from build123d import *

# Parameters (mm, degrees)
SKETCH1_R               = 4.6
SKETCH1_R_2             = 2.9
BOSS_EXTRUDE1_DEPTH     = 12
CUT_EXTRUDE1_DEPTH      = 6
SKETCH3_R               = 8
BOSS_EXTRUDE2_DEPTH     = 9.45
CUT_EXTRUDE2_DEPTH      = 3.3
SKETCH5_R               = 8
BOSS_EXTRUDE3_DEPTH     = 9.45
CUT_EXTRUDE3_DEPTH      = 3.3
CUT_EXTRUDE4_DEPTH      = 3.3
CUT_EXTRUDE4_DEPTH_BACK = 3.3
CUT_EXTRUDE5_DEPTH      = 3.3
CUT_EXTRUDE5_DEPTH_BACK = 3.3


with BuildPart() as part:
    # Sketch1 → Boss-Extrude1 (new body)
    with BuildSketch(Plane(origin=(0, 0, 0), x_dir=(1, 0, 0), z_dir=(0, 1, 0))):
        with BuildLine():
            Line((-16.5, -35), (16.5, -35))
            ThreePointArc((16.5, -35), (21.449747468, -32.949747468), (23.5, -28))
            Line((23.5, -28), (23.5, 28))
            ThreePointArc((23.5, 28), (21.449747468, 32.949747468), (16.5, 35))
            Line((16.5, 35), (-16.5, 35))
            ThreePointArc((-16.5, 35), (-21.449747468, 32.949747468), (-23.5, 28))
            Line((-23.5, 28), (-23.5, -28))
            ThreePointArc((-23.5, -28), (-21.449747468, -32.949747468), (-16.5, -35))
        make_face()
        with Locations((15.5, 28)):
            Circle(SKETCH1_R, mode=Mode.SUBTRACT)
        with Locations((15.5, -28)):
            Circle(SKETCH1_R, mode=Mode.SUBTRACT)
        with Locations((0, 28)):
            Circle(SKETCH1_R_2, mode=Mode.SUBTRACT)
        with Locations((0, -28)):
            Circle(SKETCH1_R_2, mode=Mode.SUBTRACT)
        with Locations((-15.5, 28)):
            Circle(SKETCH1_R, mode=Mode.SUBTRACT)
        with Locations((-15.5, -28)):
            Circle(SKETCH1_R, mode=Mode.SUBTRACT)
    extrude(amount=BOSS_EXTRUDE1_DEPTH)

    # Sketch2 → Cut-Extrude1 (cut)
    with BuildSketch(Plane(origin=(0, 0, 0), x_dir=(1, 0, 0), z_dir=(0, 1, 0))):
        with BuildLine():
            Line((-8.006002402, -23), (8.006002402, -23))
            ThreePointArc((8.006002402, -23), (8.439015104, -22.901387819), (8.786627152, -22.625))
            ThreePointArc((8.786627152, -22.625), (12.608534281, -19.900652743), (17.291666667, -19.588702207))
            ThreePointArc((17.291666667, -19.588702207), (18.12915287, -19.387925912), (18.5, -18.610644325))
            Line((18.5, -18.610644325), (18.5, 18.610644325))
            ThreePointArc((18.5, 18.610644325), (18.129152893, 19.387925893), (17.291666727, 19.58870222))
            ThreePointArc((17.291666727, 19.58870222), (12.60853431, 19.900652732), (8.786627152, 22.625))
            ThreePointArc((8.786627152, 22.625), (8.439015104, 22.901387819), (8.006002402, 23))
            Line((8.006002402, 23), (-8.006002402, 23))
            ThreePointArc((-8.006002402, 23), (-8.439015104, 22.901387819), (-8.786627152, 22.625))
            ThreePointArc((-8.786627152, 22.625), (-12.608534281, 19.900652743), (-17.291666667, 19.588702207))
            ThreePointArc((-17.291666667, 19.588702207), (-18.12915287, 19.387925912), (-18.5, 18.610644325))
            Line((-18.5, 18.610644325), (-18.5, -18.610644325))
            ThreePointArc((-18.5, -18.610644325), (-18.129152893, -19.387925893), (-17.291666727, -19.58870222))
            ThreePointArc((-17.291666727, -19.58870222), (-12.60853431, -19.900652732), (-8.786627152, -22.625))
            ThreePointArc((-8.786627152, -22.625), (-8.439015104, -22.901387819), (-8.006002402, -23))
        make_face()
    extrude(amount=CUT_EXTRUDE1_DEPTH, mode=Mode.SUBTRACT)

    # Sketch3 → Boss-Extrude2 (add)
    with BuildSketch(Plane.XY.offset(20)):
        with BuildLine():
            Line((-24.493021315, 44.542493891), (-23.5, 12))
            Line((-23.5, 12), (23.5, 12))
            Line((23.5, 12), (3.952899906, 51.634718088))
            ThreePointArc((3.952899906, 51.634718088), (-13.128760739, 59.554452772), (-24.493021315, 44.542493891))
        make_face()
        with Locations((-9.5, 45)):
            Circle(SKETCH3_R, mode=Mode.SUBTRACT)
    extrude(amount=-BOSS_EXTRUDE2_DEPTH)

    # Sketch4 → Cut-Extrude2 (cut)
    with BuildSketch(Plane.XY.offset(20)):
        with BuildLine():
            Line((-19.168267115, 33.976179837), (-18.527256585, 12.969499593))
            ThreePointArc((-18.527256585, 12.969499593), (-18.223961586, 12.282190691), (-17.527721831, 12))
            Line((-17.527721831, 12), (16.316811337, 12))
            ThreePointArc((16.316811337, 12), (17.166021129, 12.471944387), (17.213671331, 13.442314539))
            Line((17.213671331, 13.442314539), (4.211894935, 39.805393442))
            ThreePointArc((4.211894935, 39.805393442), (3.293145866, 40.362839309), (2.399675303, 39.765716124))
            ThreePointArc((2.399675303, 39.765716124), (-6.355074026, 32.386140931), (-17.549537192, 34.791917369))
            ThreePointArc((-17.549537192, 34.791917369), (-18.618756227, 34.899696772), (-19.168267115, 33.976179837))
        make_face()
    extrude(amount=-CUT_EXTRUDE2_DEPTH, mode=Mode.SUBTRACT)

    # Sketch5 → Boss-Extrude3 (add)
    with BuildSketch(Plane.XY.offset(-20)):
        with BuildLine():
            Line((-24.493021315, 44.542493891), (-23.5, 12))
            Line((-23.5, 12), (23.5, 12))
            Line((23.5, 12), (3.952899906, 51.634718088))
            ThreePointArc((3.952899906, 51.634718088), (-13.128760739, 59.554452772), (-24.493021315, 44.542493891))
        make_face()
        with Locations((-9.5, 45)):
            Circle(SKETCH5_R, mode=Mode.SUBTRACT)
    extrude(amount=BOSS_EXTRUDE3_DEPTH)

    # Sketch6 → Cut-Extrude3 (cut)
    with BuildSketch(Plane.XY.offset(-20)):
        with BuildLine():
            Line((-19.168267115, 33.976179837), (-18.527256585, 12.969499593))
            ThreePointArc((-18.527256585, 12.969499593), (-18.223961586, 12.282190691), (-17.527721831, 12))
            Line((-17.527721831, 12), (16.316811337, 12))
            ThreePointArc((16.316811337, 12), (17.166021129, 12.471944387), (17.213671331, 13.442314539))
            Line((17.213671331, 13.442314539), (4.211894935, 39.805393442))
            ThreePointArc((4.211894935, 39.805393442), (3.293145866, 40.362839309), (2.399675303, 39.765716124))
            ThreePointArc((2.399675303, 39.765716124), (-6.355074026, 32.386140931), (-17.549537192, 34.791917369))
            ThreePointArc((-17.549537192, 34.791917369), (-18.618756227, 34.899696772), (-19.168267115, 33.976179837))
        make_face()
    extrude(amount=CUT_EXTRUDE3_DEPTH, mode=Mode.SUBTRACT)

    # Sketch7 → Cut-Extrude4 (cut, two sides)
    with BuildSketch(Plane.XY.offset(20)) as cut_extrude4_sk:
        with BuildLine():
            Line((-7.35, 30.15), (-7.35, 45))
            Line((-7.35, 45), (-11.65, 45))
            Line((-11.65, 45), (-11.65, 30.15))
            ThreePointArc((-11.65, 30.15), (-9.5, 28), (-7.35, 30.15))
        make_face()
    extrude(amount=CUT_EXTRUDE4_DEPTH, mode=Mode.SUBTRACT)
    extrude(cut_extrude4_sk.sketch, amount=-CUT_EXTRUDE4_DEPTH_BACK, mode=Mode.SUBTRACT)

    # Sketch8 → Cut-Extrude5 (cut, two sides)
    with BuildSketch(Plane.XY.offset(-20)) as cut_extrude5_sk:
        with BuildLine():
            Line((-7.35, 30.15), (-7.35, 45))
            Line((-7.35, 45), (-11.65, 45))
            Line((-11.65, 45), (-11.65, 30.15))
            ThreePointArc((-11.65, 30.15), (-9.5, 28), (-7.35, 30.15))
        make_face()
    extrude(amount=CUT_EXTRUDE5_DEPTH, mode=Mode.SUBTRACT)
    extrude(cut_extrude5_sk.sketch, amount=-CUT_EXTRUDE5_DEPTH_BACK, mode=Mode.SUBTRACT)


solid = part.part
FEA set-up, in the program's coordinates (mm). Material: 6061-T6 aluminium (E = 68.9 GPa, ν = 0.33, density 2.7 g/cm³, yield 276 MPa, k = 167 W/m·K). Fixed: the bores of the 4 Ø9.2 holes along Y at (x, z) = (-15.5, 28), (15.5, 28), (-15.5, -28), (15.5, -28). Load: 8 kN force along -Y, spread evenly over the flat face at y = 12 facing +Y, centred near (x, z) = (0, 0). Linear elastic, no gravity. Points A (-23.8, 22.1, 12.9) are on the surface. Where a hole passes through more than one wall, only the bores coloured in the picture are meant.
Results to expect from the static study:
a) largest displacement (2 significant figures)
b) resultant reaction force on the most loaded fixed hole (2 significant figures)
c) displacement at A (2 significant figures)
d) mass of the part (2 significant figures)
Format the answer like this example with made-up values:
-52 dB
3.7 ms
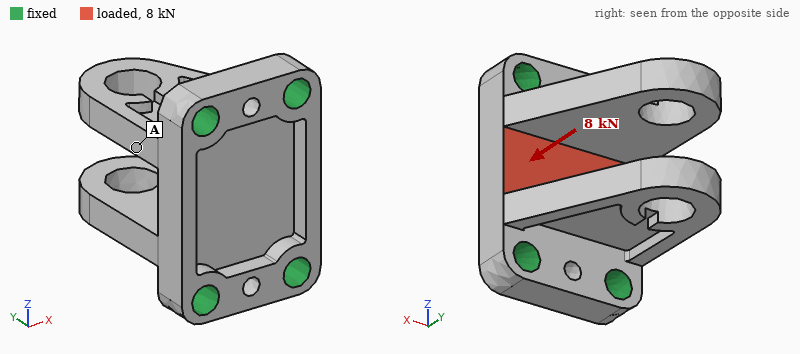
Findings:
0.12 mm
2.1 kN
0.035 mm
130 g
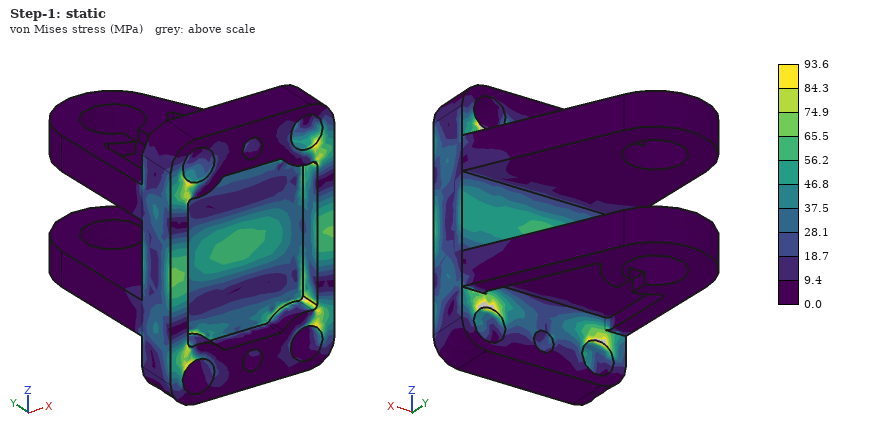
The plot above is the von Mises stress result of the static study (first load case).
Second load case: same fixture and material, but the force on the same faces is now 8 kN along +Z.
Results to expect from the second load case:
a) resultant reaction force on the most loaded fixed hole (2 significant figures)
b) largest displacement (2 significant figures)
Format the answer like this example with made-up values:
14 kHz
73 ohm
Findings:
2.1 kN
5.5 µm
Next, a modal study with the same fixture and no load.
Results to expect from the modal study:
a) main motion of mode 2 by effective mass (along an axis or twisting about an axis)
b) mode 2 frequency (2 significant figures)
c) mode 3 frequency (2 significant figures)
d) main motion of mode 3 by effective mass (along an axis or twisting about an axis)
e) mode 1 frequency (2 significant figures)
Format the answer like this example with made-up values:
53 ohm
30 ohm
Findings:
along Z
3000 Hz
6900 Hz
along X
2700 Hz
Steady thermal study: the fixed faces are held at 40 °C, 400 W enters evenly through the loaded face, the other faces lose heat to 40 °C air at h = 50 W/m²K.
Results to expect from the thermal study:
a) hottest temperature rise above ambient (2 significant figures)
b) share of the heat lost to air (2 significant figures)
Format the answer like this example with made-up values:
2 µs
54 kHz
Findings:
73 K
6.0 %
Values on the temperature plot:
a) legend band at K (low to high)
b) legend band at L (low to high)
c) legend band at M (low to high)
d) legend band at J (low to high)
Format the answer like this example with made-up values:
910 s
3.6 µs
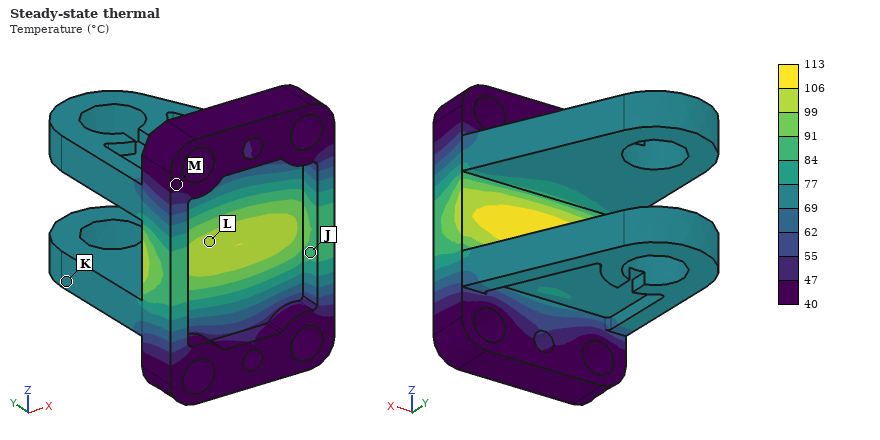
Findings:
69 to 77 °C
99 to 106 °C
40 to 47 °C
84 to 91 °C
